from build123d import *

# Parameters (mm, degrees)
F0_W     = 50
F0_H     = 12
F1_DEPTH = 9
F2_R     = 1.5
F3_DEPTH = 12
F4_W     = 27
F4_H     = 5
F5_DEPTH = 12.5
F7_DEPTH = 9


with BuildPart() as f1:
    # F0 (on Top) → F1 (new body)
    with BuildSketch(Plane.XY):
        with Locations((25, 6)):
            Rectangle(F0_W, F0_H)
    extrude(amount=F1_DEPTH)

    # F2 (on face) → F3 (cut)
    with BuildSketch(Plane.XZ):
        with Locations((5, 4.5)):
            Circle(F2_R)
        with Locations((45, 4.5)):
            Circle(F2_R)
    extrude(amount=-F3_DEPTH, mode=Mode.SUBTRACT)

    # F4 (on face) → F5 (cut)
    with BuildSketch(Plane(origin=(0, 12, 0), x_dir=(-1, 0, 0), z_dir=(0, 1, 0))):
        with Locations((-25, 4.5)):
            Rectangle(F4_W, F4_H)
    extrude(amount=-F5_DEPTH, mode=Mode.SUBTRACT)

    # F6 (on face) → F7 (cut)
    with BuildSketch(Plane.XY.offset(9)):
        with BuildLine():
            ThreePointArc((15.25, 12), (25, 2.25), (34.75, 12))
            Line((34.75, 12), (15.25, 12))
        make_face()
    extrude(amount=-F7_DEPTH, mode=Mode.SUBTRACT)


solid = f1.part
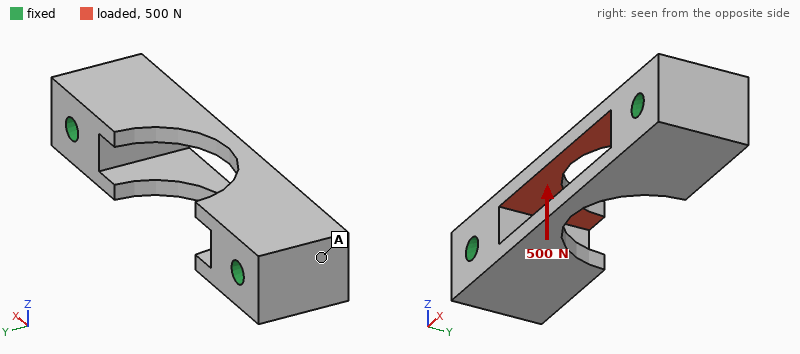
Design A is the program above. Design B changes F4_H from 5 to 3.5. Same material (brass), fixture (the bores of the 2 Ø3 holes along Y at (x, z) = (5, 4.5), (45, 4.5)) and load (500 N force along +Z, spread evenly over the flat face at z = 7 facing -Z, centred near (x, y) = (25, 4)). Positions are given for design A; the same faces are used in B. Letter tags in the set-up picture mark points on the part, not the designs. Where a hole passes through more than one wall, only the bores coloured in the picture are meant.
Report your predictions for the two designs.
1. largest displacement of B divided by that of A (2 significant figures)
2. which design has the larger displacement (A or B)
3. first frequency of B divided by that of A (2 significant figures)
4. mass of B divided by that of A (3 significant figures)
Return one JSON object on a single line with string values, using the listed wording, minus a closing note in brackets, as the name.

{"largest displacement of B divided by that of A": "0.47", "which design has the larger displacement": "A", "first frequency of B divided by that of A": "1.2", "mass of B divided by that of A": "1.09"}
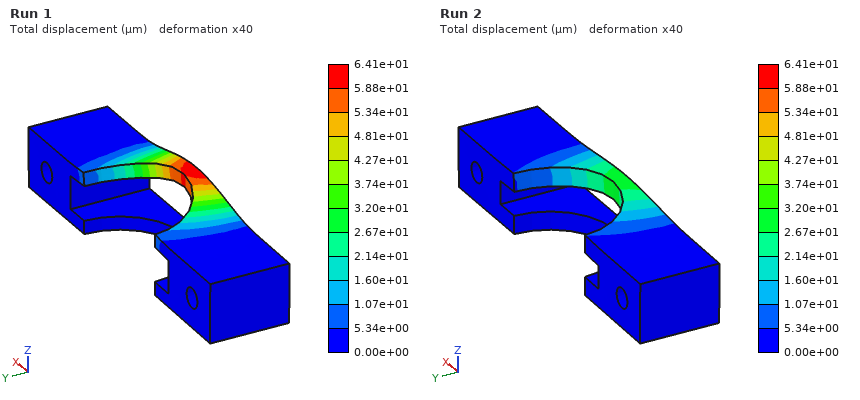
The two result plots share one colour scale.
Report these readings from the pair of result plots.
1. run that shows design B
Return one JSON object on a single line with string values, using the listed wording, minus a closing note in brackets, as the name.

{"run that shows design B": "Run 2"}
